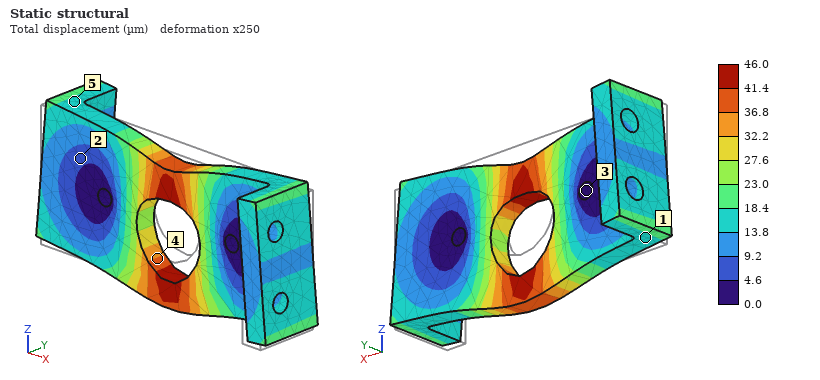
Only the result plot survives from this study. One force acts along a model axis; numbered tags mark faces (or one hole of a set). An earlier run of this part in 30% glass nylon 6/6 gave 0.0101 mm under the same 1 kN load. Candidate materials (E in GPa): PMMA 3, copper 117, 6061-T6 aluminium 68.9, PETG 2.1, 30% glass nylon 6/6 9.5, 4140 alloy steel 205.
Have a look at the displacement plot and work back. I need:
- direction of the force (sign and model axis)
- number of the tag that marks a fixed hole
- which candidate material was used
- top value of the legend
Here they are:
-Z
3
PETG
46.0 µm
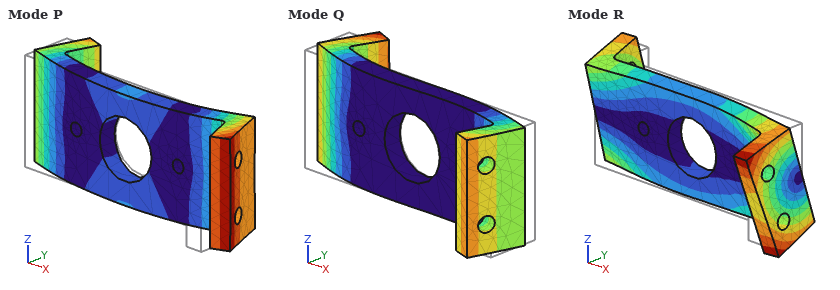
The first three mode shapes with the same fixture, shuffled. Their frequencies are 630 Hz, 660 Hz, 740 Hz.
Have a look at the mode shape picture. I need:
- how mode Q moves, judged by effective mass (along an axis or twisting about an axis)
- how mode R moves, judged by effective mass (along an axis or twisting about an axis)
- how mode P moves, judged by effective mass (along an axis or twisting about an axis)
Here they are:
twisting about Z
twisting about X
along Y
